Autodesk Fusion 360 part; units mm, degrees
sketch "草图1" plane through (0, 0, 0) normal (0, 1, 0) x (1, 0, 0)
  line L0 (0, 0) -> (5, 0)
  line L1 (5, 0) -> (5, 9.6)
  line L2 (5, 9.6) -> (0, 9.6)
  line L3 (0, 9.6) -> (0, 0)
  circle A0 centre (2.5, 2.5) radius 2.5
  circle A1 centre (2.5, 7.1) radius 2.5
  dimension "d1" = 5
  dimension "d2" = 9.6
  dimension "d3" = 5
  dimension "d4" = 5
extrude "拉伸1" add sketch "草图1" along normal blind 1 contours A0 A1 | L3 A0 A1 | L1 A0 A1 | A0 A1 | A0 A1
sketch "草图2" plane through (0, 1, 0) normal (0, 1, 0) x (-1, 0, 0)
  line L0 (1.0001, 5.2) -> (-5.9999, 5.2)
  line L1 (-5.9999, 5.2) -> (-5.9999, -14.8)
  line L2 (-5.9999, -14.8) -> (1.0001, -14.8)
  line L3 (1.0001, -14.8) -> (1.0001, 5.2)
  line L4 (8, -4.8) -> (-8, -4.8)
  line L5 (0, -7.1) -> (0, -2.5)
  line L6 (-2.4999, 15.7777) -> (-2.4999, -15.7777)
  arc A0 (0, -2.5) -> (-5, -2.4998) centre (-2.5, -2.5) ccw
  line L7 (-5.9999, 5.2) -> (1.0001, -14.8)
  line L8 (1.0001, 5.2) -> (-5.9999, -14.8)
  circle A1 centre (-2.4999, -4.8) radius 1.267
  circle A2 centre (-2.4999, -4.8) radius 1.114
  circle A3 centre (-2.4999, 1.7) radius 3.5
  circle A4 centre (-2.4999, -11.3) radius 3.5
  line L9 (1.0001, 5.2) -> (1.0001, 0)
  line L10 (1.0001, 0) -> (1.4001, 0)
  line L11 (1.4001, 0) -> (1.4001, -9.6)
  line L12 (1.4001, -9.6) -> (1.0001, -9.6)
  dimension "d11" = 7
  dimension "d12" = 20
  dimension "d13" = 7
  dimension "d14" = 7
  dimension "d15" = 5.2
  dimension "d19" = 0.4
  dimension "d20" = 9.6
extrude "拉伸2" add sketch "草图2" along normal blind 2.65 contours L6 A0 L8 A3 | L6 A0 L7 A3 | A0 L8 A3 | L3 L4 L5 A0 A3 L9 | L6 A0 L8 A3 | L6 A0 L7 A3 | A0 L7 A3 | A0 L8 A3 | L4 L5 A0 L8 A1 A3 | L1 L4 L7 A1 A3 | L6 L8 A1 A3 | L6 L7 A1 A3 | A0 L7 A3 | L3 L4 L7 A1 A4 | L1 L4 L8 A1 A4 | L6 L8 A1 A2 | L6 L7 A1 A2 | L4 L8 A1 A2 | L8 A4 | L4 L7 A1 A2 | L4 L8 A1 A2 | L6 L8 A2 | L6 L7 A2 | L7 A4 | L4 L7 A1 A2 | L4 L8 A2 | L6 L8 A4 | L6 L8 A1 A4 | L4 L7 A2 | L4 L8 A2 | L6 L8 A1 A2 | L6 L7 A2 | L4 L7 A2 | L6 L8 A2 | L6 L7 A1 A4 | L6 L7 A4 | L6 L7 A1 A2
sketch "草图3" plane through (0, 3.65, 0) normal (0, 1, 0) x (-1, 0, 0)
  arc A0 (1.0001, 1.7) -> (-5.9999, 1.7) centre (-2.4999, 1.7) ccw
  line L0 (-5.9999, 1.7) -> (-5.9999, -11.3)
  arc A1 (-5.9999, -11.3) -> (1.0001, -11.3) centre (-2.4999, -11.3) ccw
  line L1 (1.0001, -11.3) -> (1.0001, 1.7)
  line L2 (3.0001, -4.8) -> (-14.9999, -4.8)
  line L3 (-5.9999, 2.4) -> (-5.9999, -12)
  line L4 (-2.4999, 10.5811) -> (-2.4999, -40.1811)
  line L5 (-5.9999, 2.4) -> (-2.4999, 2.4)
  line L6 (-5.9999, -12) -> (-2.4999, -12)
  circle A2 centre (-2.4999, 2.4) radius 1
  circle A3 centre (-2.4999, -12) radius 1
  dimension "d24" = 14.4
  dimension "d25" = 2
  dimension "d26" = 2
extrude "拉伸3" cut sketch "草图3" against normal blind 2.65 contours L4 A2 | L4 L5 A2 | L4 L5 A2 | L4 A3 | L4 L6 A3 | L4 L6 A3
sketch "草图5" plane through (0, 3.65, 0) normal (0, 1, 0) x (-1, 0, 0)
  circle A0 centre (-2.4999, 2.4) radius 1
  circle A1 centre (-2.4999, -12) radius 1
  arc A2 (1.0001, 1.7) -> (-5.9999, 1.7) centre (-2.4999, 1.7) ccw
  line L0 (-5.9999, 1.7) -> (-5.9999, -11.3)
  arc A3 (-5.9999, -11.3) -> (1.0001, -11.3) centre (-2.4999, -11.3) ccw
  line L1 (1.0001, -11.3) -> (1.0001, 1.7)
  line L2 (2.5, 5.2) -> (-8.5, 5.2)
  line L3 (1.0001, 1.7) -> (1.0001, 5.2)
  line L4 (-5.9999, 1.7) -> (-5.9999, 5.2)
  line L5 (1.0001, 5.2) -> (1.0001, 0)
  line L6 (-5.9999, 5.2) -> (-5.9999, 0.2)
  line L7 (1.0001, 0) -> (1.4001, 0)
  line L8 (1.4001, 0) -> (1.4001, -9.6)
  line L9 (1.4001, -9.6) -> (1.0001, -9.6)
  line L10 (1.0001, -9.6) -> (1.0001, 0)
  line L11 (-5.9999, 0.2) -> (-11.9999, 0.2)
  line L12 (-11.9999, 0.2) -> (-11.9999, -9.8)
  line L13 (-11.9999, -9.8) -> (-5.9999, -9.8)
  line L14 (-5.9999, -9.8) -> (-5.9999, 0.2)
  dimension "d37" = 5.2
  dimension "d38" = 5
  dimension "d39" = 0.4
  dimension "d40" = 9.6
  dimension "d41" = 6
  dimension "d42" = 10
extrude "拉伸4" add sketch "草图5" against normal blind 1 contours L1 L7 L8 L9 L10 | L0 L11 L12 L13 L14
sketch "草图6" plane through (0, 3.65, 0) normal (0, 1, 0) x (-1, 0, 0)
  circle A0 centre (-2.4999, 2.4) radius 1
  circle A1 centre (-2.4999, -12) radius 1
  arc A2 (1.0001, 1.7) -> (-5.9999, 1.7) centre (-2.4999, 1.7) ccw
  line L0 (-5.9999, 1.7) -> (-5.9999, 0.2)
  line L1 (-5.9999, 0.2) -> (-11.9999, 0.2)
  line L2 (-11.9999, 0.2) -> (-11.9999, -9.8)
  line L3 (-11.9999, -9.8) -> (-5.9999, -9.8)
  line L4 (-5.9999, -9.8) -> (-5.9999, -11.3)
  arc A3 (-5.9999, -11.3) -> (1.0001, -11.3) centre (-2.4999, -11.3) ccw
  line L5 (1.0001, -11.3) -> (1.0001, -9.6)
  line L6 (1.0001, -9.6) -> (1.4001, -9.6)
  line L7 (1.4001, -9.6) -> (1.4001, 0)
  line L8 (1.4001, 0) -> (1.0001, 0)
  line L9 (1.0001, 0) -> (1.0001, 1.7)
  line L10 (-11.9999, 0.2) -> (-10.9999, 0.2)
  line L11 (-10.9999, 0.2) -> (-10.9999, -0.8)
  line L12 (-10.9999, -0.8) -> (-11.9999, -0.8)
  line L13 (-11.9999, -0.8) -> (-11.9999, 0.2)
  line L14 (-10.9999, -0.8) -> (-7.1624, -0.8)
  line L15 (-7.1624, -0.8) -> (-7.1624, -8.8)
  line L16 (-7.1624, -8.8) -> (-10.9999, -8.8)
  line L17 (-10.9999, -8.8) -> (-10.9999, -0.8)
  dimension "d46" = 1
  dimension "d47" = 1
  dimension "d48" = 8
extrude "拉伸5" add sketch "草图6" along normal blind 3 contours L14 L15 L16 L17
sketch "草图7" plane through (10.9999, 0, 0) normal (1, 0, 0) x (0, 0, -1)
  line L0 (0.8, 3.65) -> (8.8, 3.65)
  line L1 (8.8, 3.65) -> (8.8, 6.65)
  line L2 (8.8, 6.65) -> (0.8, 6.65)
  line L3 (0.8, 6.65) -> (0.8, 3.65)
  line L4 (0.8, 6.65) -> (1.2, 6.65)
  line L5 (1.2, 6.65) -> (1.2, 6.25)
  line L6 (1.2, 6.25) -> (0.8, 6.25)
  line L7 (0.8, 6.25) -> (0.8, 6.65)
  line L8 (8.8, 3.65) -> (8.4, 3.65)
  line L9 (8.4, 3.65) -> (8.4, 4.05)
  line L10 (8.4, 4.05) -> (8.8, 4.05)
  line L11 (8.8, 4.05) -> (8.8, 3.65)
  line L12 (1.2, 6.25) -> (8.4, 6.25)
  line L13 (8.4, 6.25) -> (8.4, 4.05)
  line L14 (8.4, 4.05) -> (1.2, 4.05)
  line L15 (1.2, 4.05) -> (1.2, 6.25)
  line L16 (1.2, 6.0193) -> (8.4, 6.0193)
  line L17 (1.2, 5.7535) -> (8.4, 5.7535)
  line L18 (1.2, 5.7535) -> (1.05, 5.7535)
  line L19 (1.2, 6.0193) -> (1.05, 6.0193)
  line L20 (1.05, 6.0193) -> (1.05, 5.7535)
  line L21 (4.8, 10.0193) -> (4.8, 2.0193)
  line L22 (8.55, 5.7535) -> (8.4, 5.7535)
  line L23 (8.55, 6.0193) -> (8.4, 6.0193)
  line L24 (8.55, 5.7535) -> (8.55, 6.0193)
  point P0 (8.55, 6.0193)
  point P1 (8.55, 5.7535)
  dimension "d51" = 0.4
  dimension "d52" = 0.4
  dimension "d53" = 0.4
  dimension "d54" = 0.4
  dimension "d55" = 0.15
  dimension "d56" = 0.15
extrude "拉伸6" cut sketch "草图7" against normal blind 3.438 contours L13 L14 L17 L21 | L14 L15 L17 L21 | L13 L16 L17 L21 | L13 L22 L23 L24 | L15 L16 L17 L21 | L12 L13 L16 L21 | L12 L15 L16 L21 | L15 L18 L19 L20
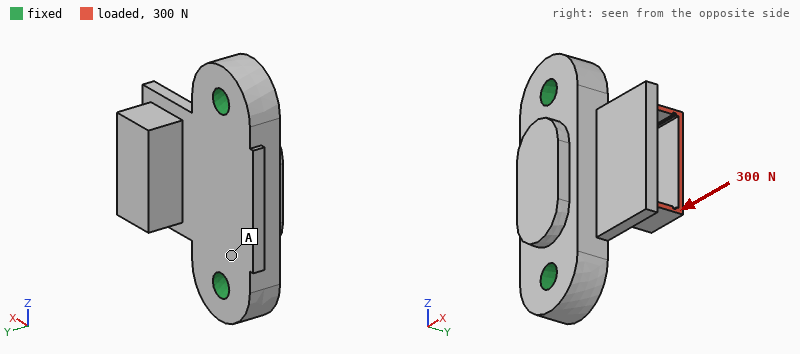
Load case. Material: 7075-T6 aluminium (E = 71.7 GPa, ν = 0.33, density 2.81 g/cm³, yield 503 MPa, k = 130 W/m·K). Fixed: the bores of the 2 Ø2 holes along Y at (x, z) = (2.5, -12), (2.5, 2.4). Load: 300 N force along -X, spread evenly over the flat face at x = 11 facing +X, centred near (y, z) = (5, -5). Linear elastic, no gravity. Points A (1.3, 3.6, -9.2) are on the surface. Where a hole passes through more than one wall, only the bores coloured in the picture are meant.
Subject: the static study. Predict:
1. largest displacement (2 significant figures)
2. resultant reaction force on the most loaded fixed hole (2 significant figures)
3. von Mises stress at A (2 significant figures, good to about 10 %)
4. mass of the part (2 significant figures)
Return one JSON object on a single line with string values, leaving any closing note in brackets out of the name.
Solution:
{"largest displacement": "0.16 mm", "resultant reaction force on the most loaded fixed hole": "160 N", "von Mises stress at A": "41 MPa", "mass of the part": "1.3 g"}
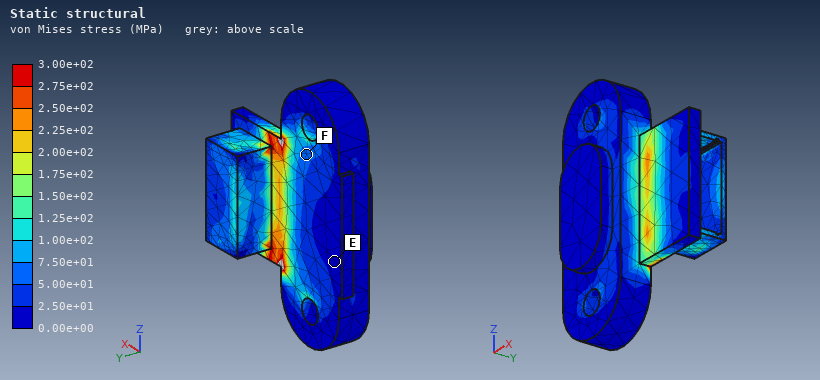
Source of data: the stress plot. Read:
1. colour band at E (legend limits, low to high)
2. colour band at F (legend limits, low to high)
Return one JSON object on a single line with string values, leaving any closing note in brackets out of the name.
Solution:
{"colour band at E": "0.00e+00 to 2.50e+01 MPa", "colour band at F": "5.00e+01 to 7.50e+01 MPa"}
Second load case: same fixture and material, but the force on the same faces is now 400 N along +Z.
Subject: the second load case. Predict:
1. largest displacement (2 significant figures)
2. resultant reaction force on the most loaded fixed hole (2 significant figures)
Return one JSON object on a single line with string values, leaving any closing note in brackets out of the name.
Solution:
{"largest displacement": "61 µm", "resultant reaction force on the most loaded fixed hole": "330 N"}
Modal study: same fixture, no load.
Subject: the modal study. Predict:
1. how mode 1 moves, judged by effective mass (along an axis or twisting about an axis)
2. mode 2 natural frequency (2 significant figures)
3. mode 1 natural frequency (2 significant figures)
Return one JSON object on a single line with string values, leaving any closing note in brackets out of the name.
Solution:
{"how mode 1 moves, judged by effective mass": "along Y", "mode 2 natural frequency": "33 kHz", "mode 1 natural frequency": "14 kHz"}
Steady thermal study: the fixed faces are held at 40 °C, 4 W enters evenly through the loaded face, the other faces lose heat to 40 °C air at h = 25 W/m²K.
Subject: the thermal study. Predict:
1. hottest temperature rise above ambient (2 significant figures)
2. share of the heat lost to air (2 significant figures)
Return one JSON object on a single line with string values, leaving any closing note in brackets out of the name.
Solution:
{"hottest temperature rise above ambient": "29 K", "share of the heat lost to air": "3.1 %"}
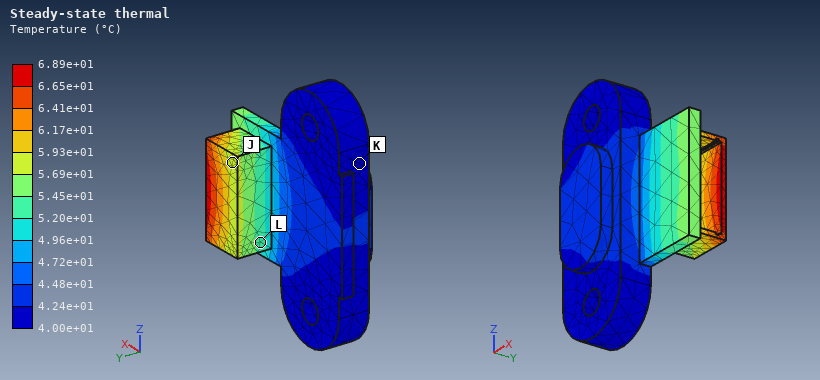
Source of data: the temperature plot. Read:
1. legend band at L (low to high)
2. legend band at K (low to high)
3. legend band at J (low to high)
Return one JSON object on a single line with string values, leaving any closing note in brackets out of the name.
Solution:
{"legend band at L": "5.20e+01 to 5.45e+01 °C", "legend band at K": "4.00e+01 to 4.24e+01 °C", "legend band at J": "5.69e+01 to 5.93e+01 °C"}
